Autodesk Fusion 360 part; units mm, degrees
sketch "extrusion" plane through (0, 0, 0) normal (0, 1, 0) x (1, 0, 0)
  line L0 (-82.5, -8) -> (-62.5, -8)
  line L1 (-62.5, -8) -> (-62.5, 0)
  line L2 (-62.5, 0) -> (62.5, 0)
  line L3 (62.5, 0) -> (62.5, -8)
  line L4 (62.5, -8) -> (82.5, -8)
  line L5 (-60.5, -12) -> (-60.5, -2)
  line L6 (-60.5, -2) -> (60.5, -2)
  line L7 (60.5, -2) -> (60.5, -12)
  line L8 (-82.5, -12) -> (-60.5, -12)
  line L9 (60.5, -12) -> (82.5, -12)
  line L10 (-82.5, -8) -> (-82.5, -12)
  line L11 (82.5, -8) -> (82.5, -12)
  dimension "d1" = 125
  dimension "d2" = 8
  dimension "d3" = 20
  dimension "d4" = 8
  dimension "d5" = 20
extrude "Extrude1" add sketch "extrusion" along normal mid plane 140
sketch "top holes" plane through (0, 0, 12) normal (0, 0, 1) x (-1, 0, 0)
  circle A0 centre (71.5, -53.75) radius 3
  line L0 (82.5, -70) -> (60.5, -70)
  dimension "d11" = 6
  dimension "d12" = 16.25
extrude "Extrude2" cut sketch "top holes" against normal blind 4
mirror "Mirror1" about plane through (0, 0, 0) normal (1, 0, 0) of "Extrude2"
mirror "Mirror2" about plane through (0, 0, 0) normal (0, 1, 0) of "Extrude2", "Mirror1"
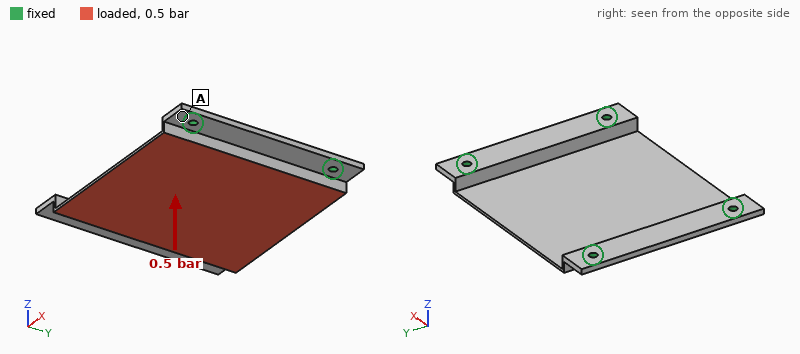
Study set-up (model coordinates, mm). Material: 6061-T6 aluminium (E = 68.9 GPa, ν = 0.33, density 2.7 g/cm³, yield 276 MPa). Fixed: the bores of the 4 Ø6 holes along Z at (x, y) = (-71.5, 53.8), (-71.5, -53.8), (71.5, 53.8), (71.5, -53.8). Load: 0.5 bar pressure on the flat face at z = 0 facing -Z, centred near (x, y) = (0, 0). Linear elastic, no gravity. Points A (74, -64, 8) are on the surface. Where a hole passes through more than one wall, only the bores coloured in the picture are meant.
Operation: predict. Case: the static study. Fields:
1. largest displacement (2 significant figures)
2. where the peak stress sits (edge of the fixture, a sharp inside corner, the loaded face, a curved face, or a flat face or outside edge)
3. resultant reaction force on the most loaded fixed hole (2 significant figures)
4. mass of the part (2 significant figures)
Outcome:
0.72 mm
the loaded face
710 N
170 g
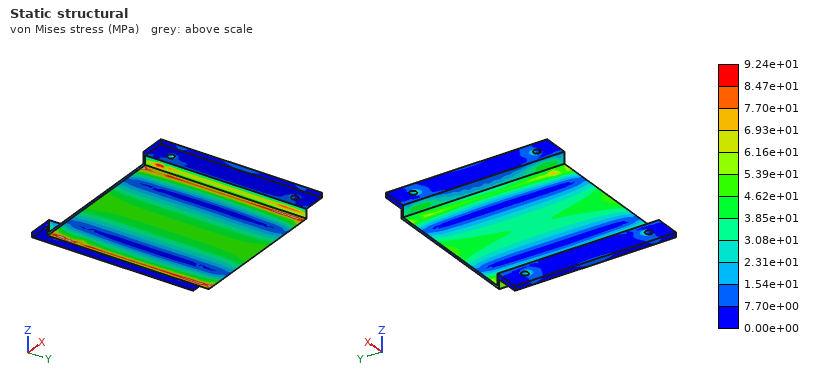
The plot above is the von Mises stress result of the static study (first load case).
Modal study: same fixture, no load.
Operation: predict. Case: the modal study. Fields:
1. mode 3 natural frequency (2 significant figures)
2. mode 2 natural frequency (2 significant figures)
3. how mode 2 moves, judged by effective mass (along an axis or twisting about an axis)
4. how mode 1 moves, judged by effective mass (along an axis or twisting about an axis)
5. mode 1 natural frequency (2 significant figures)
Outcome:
1200 Hz
790 Hz
twisting about X
along Z
680 Hz
